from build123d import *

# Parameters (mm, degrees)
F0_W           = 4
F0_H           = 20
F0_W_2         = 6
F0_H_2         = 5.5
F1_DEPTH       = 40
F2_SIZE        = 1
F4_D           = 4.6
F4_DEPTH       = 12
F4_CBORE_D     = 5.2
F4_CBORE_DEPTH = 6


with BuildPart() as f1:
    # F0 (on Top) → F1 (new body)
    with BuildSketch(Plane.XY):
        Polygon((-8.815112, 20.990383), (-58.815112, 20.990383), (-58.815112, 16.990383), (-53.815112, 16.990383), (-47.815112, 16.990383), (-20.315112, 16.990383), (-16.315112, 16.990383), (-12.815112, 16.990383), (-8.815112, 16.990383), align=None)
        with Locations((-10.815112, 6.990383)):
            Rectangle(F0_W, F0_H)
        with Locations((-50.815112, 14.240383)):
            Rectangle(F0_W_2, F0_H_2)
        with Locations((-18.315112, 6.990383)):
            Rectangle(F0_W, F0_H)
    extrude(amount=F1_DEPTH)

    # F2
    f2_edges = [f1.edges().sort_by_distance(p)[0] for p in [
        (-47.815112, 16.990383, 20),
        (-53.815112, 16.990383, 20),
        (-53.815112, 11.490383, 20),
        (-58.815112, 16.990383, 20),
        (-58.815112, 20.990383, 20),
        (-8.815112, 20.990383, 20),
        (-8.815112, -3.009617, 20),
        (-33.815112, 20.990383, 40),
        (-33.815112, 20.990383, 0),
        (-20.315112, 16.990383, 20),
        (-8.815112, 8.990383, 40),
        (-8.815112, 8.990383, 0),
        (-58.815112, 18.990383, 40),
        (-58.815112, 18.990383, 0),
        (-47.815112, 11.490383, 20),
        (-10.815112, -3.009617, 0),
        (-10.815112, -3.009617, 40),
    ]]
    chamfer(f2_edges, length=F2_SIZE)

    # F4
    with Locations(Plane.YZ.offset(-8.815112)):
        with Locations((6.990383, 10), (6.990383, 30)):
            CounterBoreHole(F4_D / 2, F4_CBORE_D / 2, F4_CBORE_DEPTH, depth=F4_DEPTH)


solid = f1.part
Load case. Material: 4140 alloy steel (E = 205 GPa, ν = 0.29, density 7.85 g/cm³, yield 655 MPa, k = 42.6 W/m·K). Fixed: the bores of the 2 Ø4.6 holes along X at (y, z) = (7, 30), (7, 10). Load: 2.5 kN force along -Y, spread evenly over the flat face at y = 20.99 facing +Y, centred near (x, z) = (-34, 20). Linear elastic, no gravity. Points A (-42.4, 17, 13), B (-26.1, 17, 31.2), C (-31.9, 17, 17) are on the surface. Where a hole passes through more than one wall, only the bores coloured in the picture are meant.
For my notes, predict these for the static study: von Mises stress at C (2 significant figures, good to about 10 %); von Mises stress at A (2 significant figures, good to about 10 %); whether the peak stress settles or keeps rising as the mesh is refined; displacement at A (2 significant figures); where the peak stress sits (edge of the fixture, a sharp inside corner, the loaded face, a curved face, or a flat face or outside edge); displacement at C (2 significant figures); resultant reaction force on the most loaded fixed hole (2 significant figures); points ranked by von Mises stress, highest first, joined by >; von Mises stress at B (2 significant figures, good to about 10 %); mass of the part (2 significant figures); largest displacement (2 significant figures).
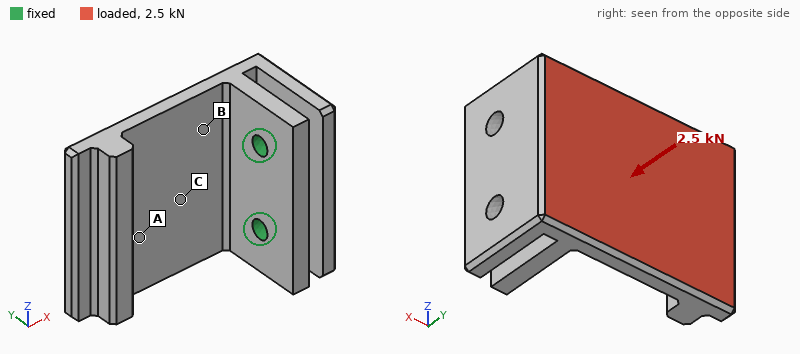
150 MPa
56 MPa
keeps rising
0.36 mm
edge of the fixture
0.17 mm
1.3 kN
B > C > A
220 MPa
120 g
0.67 mm
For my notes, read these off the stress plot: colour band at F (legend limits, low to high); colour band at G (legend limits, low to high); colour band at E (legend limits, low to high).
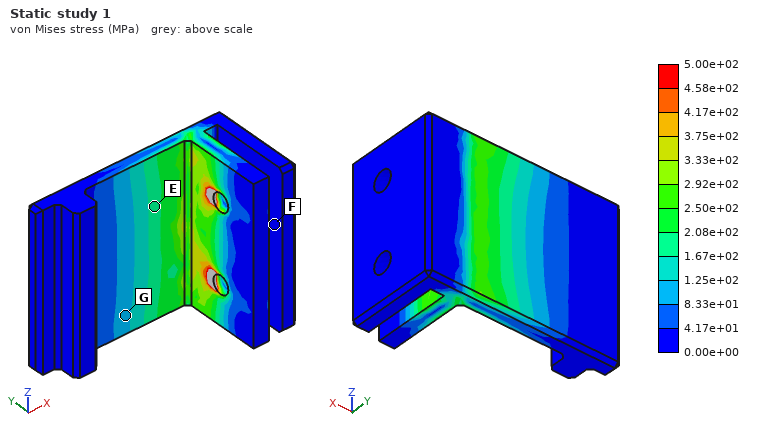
0.00e+00 to 4.17e+01 MPa
8.33e+01 to 1.25e+02 MPa
1.67e+02 to 2.08e+02 MPa
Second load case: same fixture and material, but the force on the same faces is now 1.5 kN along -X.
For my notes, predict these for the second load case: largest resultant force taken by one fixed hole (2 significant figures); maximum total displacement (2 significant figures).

750 N
0.15 mm
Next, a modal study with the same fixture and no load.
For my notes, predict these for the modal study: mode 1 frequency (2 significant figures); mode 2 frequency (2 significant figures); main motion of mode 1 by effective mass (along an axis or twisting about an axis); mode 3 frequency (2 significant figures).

1200 Hz
3100 Hz
along Y
4300 Hz
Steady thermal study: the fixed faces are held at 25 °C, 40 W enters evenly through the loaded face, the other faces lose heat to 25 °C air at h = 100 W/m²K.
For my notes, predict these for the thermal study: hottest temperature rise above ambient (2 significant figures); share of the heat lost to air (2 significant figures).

70 K
55 %
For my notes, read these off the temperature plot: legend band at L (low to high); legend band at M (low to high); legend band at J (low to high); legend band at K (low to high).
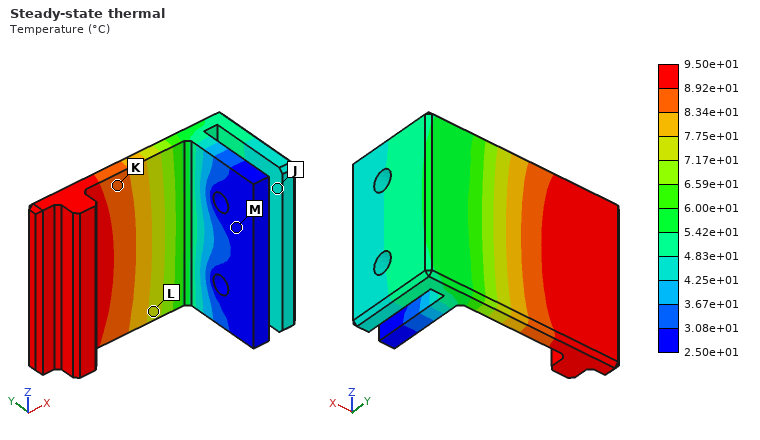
7.17e+01 to 7.75e+01 °C
2.50e+01 to 3.08e+01 °C
4.25e+01 to 4.83e+01 °C
8.34e+01 to 8.92e+01 °C
